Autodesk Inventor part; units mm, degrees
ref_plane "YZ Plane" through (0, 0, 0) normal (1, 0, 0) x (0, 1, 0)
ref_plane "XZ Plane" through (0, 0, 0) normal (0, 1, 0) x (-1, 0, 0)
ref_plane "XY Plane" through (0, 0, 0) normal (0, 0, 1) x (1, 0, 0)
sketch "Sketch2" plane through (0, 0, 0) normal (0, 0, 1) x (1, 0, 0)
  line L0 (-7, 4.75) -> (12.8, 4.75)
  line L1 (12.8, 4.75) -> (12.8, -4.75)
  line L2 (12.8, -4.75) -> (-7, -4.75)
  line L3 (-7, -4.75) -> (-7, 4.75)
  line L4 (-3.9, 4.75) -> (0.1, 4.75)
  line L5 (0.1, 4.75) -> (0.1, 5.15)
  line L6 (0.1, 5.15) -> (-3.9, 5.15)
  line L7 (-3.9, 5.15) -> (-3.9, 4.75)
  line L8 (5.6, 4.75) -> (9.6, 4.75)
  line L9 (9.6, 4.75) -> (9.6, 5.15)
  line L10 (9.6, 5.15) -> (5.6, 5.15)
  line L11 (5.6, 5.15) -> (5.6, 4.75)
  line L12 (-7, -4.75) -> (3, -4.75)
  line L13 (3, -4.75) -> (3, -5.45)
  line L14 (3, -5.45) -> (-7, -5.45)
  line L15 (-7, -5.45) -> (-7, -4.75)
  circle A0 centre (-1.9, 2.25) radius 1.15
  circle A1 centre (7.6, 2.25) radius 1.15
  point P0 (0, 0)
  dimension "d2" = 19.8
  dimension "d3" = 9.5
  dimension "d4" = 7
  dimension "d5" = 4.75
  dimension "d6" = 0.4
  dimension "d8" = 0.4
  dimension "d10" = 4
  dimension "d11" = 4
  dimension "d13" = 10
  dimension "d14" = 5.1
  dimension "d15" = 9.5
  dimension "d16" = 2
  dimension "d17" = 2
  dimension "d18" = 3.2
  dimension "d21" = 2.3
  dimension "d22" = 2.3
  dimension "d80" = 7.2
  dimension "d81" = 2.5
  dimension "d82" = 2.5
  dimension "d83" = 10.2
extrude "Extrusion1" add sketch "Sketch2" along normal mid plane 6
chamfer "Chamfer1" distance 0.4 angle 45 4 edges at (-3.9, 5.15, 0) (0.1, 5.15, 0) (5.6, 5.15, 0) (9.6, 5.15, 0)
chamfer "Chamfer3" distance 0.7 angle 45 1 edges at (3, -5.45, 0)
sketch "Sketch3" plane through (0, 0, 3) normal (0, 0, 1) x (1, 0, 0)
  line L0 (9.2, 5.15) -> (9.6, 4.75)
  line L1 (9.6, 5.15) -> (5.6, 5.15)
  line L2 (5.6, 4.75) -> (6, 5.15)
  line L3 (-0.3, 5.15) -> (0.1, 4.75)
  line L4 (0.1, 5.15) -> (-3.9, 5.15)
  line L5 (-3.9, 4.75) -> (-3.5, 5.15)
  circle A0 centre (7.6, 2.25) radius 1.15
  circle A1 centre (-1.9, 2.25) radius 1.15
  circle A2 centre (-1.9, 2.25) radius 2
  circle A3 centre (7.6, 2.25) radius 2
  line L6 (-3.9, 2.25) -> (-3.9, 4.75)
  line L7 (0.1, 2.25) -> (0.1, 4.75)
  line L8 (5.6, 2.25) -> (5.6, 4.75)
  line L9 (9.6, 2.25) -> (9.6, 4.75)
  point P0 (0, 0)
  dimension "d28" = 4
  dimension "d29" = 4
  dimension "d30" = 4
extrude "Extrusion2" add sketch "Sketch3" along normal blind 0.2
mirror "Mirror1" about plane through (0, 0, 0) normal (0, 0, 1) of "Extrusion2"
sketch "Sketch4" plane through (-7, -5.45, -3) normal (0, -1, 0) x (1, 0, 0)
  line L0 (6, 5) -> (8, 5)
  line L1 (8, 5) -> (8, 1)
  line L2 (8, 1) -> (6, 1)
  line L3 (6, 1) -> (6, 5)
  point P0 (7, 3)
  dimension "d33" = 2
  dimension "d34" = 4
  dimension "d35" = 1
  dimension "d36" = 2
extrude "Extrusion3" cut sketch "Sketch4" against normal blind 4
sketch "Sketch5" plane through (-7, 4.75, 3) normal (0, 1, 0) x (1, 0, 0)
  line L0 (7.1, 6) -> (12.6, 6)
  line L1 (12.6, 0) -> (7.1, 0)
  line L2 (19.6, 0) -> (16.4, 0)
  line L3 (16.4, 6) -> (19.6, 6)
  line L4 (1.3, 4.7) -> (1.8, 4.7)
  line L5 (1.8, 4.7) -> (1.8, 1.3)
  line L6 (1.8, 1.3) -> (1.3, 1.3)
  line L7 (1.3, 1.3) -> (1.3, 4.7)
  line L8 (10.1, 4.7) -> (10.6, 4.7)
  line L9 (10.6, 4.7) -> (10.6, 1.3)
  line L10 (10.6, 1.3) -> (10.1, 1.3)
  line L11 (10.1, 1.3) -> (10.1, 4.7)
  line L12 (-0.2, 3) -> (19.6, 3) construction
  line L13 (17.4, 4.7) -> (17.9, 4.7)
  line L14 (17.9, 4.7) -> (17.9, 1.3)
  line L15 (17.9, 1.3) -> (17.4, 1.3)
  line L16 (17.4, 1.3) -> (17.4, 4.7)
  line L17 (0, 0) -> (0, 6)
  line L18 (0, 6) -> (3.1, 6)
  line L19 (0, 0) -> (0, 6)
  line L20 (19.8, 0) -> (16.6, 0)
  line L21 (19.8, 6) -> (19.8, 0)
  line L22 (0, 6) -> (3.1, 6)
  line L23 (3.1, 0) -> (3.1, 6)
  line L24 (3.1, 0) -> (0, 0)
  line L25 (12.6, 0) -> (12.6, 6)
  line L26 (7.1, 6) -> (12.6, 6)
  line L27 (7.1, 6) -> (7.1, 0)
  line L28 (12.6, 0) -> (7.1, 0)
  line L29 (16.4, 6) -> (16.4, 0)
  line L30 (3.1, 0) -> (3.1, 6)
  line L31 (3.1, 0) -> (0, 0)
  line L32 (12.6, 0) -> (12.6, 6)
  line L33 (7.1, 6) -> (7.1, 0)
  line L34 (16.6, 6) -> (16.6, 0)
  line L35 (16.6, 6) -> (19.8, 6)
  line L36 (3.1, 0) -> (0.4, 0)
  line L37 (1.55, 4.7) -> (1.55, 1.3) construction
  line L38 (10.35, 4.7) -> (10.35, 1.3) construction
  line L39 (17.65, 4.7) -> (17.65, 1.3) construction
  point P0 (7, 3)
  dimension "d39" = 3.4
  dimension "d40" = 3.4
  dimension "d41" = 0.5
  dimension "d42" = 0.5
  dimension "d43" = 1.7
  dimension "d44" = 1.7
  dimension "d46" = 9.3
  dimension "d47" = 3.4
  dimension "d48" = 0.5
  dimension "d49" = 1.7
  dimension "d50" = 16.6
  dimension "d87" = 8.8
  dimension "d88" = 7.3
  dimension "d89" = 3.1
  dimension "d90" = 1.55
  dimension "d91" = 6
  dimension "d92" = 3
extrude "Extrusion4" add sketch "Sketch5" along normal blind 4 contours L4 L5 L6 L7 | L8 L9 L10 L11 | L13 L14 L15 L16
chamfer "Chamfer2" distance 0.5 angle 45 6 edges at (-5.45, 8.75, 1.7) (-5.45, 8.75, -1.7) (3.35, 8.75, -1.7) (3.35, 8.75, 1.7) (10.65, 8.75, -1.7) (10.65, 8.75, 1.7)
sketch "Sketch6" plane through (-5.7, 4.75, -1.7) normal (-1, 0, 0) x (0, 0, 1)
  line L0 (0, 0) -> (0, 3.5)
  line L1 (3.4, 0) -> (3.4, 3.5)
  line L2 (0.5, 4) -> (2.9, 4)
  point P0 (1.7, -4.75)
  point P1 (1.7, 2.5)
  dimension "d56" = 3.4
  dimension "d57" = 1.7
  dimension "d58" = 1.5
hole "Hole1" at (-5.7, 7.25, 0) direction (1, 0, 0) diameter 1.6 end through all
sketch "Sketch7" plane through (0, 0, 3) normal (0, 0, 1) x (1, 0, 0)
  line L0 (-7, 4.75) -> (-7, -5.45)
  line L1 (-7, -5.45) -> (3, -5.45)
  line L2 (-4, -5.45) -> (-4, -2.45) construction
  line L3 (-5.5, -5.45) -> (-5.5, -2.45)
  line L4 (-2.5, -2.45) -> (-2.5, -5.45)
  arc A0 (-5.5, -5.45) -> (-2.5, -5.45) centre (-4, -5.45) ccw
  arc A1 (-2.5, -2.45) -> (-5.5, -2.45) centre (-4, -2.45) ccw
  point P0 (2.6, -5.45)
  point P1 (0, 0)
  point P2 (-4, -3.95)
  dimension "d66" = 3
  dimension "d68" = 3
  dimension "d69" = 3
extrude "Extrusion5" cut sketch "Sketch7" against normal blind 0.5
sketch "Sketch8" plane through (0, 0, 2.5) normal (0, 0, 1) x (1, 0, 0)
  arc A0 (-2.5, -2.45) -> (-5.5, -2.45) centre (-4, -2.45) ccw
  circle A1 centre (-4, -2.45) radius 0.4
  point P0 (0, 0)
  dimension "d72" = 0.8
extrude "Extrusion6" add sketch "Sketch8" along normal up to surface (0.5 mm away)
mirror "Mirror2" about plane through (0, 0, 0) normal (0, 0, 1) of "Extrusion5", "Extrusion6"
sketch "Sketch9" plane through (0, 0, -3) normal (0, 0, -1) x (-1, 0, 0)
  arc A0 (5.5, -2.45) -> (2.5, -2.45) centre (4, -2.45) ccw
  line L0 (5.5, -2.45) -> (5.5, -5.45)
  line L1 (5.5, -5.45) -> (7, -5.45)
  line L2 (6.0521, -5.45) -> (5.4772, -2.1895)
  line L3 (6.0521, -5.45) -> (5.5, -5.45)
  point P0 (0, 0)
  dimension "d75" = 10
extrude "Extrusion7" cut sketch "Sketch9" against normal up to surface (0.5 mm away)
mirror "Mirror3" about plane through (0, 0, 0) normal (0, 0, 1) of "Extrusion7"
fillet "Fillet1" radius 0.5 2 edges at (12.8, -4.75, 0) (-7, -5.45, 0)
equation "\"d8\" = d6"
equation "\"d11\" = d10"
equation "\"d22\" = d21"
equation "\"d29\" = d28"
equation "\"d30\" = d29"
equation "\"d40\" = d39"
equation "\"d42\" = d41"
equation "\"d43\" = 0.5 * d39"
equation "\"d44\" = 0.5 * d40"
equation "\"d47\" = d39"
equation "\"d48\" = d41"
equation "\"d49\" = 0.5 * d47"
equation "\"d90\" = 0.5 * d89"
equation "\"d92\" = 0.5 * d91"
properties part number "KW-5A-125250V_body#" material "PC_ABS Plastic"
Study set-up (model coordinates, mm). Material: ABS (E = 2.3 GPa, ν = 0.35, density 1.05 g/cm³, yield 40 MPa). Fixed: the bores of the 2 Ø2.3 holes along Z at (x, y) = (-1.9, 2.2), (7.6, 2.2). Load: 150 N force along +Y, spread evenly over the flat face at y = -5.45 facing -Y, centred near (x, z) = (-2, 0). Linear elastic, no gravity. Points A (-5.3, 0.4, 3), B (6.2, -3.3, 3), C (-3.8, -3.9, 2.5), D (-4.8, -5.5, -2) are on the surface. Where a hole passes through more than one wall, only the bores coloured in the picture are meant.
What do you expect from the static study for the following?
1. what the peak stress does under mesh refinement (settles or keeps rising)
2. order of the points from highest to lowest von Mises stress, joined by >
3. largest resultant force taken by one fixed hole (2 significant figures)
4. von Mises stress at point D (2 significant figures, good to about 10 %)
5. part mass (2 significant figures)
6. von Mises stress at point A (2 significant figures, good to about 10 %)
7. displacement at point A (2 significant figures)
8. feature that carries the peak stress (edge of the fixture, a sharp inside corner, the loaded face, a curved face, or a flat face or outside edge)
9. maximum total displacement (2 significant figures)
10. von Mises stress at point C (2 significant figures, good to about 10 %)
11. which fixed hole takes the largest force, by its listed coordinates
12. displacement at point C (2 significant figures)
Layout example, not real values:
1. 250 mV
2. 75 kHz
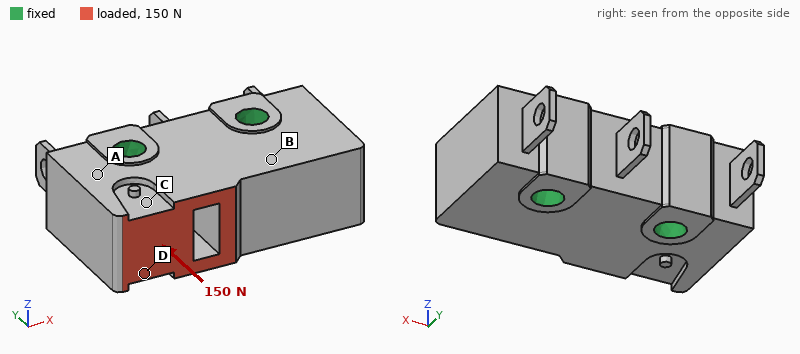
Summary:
1. keeps rising
2. C > D > A > B
3. 140 N
4. 3.3 MPa
5. 1.2 g
6. 2.1 MPa
7. 9.8 µm
8. edge of the fixture
9. 20 µm
10. 4.0 MPa
11. (-1.9, 2.2)
12. 15 µm
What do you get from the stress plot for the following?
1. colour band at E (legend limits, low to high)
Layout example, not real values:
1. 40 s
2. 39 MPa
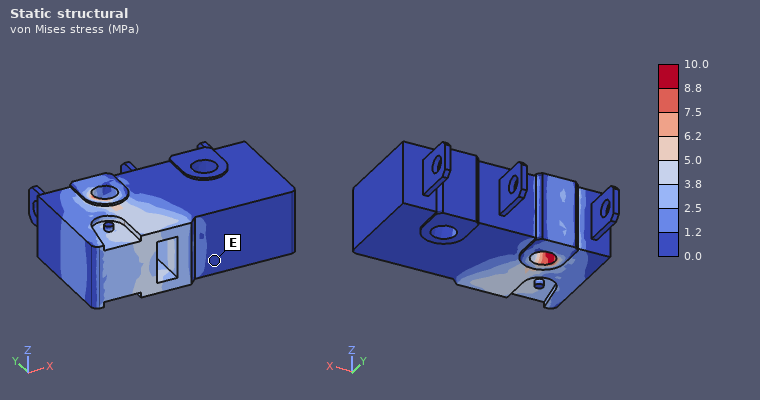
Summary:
1. 0.0 to 1.2 MPa
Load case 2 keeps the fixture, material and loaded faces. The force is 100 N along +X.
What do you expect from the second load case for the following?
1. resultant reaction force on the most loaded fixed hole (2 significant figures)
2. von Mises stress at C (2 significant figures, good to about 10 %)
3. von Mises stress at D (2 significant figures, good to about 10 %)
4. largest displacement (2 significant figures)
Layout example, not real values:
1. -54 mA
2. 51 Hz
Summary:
1. 80 N
2. 5.0 MPa
3. 4.9 MPa
4. 44 µm
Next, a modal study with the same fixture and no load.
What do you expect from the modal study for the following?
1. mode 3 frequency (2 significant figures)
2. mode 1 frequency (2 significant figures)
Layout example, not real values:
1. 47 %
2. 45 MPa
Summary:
1. 7800 Hz
2. 7800 Hz
